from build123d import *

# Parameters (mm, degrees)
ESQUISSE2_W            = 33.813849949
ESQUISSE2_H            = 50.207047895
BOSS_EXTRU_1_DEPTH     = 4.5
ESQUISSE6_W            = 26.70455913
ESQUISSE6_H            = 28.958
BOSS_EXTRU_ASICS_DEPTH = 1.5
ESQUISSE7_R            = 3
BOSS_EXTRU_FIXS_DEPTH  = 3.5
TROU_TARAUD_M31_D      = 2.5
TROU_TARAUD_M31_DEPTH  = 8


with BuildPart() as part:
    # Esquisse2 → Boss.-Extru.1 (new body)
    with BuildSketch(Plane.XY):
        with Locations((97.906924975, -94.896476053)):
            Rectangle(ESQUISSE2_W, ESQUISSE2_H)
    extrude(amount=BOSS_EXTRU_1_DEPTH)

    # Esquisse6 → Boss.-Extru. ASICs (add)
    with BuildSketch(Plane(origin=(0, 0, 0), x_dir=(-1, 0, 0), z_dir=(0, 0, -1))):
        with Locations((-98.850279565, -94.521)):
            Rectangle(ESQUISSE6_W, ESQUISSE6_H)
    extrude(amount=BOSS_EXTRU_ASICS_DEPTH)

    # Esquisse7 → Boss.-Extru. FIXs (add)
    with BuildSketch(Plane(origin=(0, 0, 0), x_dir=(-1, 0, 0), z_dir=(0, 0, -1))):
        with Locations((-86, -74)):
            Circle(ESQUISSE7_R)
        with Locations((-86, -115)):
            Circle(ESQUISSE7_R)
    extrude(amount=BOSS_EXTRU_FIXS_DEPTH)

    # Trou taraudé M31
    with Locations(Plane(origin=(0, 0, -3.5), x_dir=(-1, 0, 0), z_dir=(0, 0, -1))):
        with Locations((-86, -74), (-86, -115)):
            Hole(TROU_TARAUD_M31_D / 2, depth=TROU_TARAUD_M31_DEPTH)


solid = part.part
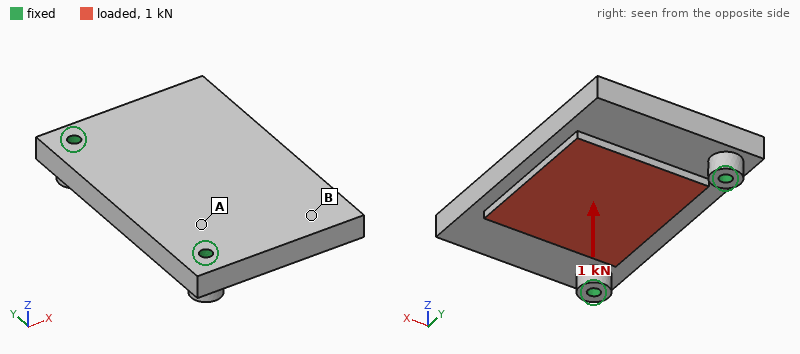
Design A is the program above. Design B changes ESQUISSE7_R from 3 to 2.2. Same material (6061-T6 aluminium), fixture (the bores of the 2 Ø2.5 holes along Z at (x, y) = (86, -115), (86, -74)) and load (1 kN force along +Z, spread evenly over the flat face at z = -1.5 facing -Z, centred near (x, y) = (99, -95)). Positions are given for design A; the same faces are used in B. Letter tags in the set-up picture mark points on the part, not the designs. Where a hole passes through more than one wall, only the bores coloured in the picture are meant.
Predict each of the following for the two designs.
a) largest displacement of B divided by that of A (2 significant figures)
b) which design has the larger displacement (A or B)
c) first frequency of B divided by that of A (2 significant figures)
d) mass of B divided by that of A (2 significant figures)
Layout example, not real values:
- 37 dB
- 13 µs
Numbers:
- 1.1
- B
- 0.95
- 0.99
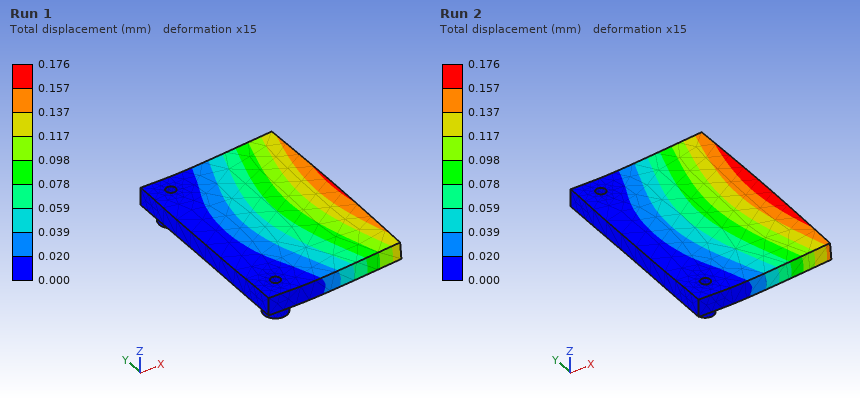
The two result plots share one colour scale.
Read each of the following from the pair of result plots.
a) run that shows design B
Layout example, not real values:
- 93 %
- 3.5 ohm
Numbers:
- Run 2
